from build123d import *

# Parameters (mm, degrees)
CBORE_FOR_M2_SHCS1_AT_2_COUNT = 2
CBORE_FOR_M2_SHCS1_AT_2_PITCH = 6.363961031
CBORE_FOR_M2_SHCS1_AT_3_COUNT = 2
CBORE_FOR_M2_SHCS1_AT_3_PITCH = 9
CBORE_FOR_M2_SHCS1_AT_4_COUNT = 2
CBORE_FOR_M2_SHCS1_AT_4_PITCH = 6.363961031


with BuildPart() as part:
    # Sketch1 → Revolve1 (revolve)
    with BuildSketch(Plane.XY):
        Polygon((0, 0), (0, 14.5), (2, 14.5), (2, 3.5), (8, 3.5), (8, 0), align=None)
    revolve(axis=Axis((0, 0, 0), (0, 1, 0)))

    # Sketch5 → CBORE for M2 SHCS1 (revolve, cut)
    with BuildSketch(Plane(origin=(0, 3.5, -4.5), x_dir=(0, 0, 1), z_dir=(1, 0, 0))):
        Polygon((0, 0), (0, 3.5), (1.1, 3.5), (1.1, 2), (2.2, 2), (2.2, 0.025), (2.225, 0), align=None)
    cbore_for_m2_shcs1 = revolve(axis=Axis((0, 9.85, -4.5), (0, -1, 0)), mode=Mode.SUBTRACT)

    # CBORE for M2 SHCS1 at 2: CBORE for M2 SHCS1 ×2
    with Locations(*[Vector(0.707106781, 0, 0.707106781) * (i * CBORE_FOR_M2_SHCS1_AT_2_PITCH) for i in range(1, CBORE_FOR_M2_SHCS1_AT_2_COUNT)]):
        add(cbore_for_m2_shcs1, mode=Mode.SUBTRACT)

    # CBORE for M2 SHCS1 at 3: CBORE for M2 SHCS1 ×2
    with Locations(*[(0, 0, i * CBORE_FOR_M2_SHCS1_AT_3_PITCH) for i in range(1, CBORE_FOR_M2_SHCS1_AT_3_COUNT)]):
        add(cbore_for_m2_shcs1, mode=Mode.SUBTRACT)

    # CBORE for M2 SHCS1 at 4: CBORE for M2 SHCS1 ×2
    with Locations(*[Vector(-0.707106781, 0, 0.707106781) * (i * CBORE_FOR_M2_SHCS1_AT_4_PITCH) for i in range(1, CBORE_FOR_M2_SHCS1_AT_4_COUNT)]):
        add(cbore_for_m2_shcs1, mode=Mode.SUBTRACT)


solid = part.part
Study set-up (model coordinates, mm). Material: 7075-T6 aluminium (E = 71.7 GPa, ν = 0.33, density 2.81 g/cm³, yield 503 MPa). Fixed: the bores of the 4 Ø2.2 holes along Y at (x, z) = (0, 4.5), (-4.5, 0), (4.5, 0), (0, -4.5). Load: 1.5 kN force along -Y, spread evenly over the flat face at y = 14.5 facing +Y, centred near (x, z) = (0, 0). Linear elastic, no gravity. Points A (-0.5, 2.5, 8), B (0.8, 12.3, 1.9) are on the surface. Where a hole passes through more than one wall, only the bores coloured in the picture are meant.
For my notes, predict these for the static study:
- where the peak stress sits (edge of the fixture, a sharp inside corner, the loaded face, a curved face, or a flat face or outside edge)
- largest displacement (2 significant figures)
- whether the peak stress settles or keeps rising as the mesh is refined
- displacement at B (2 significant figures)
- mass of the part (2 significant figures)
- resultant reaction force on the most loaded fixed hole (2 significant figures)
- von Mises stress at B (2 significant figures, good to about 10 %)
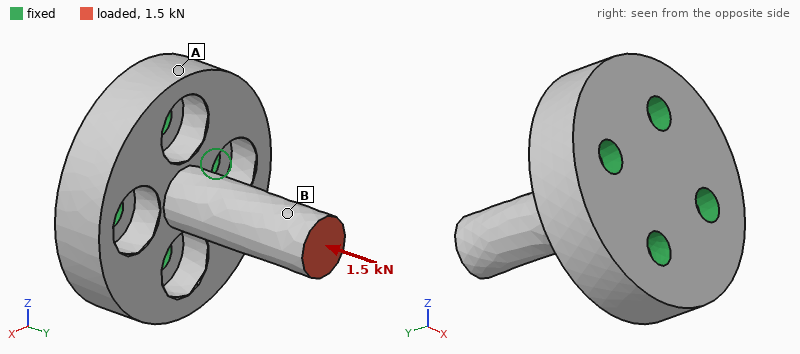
edge of the fixture
25 µm
keeps rising
21 µm
2.0 g
410 N
120 MPa
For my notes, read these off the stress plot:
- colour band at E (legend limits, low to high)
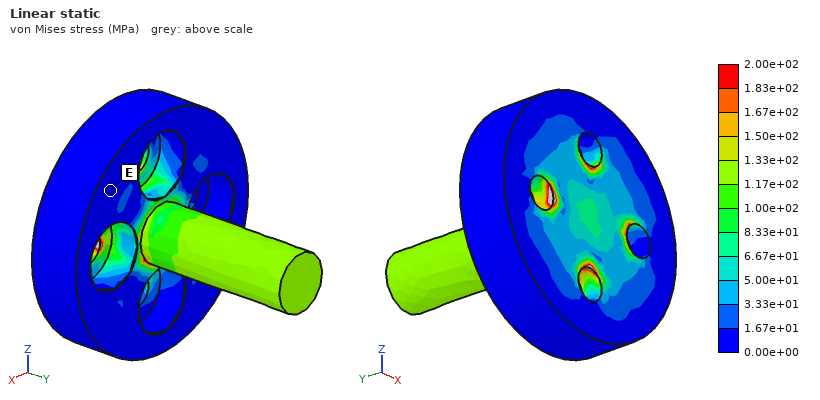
0.00e+00 to 1.67e+01 MPa
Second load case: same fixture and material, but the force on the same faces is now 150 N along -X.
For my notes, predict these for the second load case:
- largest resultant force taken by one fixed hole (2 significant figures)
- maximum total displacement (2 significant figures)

230 N
0.11 mm
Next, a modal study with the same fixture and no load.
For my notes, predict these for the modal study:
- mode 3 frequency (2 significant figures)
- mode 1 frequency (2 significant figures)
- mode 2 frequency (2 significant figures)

65 kHz
18 kHz
18 kHz
